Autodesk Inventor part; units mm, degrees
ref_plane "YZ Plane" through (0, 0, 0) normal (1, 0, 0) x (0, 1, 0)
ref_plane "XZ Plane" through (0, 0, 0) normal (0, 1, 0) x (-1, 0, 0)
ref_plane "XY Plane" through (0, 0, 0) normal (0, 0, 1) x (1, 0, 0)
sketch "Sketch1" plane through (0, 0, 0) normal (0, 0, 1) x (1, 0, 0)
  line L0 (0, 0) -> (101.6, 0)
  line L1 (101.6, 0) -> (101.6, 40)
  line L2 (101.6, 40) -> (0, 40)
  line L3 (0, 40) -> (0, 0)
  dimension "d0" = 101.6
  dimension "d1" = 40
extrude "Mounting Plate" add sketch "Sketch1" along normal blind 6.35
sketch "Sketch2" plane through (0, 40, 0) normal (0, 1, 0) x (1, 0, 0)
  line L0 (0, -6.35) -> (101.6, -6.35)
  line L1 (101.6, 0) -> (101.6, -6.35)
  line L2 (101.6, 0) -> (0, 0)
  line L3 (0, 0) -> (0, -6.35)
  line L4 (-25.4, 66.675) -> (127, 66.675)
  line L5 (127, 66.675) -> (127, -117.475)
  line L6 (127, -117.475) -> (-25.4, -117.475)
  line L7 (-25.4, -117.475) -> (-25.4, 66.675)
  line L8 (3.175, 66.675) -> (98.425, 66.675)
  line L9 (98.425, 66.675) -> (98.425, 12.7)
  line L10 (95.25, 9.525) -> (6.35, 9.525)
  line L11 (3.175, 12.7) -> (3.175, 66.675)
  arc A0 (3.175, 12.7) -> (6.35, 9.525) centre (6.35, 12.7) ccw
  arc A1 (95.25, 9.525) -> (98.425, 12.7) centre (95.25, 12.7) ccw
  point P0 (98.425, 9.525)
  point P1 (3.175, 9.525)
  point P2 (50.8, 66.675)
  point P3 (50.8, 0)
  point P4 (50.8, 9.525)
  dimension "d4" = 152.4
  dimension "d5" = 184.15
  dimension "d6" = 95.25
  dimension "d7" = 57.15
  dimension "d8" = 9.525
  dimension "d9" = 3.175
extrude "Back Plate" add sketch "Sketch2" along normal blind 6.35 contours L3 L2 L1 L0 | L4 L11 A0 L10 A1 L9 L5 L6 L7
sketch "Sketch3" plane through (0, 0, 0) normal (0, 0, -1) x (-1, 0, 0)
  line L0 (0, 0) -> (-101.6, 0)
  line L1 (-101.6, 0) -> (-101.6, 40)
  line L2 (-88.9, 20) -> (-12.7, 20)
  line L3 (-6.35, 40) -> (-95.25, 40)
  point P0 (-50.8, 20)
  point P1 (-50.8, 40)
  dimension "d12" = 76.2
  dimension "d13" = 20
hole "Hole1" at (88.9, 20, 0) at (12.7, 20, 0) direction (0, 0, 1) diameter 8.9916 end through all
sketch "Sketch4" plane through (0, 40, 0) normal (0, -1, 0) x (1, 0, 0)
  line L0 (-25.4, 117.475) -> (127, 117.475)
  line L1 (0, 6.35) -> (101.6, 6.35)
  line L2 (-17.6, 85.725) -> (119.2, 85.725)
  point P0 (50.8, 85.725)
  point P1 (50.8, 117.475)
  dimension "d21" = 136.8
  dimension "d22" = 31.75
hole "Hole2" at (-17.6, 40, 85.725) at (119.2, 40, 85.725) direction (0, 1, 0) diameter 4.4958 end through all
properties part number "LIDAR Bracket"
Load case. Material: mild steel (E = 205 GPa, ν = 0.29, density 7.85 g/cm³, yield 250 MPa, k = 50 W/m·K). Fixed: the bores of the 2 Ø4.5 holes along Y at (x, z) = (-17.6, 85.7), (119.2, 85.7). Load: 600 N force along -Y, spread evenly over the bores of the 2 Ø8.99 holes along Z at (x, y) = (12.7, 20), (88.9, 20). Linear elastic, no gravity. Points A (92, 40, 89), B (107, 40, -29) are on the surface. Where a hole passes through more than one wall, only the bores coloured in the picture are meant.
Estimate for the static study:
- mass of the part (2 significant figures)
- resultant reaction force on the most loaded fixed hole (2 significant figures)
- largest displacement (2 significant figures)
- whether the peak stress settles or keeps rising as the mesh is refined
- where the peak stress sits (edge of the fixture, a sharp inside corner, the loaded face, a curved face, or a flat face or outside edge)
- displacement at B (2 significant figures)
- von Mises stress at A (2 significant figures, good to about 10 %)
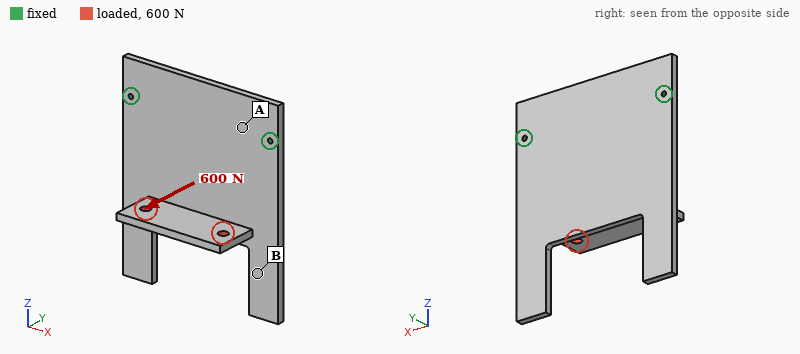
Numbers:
1.3 kg
300 N
0.65 mm
keeps rising
edge of the fixture
0.46 mm
29 MPa
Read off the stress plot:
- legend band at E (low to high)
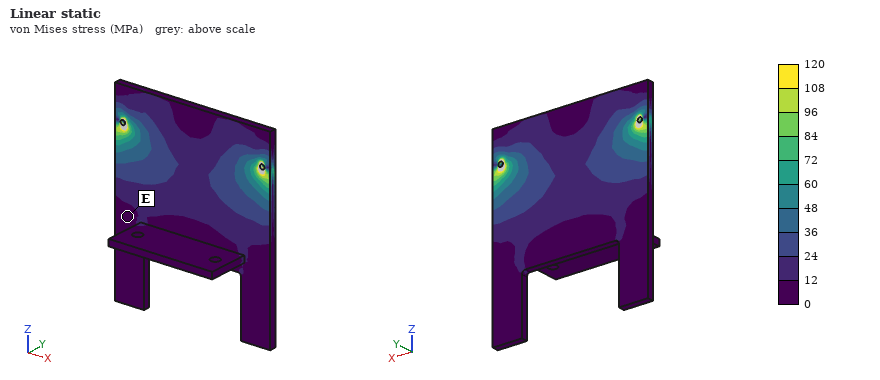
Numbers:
0 to 12 MPa
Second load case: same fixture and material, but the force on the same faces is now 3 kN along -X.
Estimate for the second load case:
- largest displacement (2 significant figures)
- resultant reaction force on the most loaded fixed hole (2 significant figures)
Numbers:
0.35 mm
2.4 kN
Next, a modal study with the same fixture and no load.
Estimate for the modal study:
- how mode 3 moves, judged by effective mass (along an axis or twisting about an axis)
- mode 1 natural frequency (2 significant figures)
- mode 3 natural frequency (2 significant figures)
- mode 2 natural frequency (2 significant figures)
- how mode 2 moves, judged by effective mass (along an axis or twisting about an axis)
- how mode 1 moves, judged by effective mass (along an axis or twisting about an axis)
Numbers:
along Y
220 Hz
1100 Hz
490 Hz
twisting about Z
along Y
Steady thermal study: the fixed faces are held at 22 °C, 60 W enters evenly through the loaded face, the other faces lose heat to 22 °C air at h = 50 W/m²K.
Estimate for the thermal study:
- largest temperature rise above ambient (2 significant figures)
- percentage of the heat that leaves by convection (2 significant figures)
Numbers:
80 K
90 %
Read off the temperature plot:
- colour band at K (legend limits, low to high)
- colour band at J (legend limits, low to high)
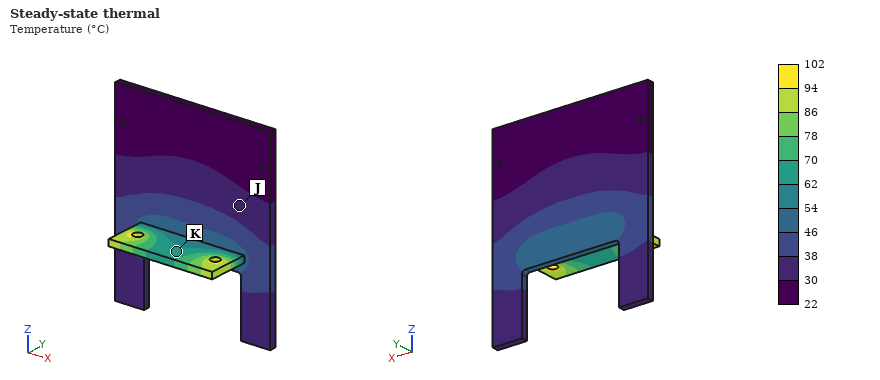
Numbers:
62 to 70 °C
30 to 38 °C
